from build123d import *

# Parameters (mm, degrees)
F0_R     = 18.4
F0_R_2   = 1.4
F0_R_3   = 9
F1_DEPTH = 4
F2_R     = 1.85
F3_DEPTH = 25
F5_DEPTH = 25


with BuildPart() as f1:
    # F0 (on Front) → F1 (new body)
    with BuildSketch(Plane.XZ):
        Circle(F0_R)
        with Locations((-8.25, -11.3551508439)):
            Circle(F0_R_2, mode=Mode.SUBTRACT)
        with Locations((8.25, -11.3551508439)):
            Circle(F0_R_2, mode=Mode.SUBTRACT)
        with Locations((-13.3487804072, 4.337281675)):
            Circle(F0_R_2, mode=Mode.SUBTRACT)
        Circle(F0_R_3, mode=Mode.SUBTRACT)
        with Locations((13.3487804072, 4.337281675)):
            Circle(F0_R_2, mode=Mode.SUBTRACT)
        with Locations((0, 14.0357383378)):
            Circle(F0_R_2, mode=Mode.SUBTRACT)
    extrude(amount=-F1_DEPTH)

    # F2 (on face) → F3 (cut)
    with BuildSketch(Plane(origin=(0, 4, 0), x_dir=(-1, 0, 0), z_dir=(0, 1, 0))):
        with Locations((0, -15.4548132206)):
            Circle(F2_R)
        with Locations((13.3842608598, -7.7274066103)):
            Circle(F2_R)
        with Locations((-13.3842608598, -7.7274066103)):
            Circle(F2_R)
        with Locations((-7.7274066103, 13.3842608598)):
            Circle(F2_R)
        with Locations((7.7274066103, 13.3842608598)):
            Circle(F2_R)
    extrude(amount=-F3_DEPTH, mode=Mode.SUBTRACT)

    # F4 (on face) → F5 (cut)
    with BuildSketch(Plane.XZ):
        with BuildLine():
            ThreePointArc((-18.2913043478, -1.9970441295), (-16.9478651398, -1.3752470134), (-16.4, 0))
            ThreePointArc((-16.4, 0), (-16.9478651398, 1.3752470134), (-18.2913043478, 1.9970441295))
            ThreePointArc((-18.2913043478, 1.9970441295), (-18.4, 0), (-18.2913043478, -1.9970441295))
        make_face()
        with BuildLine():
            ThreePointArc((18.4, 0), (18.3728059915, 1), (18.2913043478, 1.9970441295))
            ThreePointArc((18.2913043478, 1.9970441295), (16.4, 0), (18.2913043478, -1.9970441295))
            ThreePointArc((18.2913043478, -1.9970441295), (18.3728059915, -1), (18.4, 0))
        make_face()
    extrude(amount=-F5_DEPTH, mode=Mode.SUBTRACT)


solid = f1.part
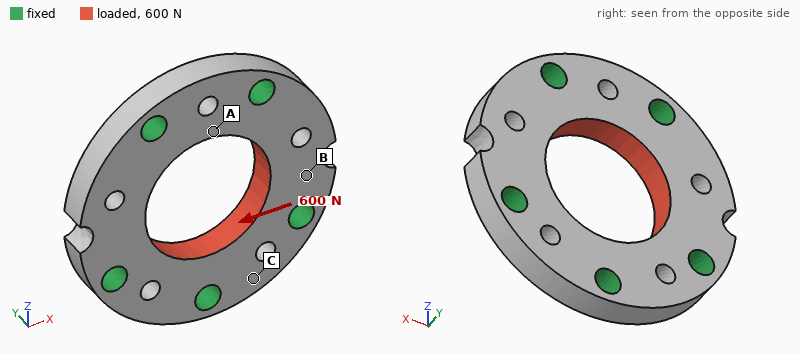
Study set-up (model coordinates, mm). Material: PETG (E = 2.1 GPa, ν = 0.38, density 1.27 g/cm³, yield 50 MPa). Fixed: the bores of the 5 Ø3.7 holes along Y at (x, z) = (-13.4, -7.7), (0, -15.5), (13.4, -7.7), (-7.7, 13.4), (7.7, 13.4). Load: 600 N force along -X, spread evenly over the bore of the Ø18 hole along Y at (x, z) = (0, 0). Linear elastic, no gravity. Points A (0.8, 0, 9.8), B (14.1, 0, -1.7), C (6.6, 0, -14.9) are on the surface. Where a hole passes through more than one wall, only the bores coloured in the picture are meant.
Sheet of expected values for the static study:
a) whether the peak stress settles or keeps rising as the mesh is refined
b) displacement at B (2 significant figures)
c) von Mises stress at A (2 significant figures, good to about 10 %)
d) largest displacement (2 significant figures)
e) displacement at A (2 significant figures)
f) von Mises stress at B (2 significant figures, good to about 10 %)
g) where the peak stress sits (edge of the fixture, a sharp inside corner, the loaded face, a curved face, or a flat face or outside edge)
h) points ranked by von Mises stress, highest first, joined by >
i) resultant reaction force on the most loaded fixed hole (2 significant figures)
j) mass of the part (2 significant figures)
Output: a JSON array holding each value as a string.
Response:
["keeps rising", "22 µm", "5.5 MPa", "36 µm", "12 µm", "3.8 MPa", "edge of the fixture", "A > B > C", "140 N", "3.6 g"]
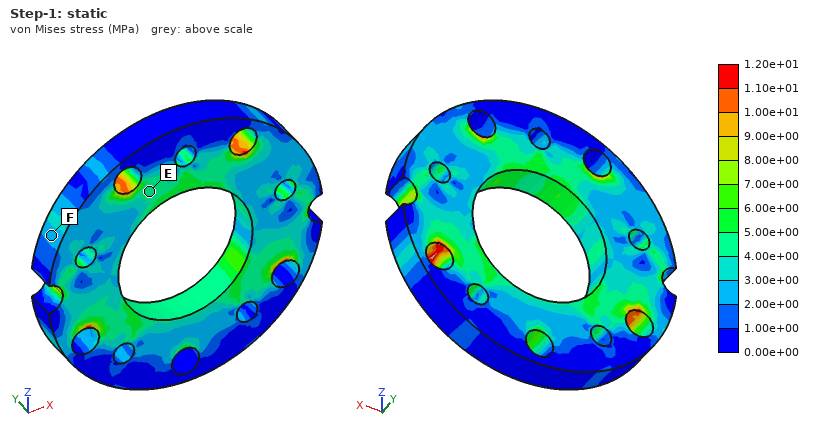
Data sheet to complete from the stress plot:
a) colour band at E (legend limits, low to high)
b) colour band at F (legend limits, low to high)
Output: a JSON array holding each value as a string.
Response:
["4.00e+00 to 5.00e+00 MPa", "2.00e+00 to 3.00e+00 MPa"]
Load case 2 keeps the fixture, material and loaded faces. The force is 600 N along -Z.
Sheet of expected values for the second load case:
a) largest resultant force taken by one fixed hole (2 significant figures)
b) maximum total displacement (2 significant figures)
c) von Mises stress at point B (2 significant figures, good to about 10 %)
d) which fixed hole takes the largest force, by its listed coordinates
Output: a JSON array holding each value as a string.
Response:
["150 N", "17 µm", "1.5 MPa", "(0, -15.5)"]
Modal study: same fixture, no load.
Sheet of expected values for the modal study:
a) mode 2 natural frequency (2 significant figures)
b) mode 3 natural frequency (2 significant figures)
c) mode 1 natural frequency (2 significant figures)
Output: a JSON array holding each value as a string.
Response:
["9100 Hz", "15 kHz", "9100 Hz"]
